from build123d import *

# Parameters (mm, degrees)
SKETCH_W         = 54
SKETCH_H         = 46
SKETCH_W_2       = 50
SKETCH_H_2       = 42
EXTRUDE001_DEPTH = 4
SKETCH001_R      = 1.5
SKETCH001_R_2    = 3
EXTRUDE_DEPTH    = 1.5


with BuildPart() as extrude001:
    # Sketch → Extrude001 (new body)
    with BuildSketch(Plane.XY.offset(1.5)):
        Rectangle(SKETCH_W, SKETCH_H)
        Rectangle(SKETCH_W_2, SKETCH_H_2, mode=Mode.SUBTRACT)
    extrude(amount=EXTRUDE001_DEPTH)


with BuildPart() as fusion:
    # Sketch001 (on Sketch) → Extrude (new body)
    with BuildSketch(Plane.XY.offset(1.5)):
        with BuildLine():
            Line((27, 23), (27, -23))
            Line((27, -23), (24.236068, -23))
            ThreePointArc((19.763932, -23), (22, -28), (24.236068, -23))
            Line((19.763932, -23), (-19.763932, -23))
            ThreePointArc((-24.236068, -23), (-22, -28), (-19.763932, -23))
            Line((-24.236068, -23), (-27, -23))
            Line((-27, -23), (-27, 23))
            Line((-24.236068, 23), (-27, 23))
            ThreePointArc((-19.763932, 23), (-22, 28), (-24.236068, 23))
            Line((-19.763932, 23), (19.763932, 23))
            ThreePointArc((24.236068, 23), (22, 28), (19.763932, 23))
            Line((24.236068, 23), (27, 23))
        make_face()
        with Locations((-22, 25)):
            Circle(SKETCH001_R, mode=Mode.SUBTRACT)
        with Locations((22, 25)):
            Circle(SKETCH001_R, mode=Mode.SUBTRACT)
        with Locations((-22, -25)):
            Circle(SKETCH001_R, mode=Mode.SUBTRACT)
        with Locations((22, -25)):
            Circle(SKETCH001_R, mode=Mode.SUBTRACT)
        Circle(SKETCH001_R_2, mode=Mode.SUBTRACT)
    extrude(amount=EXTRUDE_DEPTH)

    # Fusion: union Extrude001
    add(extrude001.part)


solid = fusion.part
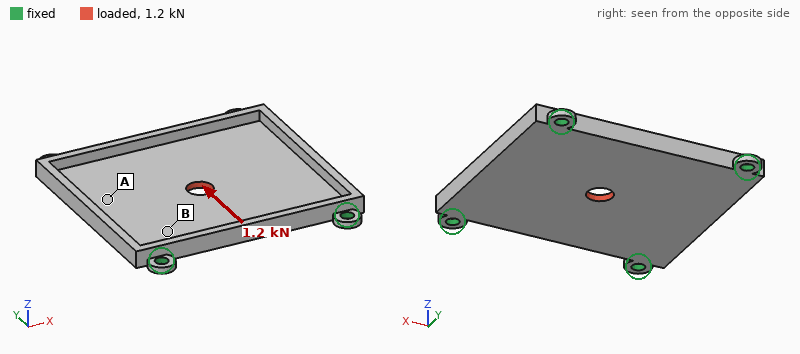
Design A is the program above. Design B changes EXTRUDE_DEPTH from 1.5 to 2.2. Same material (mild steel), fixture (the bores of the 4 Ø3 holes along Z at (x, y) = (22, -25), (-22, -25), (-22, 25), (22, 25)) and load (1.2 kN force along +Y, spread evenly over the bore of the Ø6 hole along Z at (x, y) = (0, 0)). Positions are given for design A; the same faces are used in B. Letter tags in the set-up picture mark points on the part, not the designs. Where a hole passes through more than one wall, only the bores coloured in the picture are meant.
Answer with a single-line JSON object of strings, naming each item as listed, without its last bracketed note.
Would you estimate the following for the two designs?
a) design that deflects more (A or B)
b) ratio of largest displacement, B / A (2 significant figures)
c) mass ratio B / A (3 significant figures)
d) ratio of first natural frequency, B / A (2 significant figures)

{"design that deflects more": "A", "ratio of largest displacement, B / A": "0.69", "mass ratio B / A": "1.32", "ratio of first natural frequency, B / A": "1.2"}
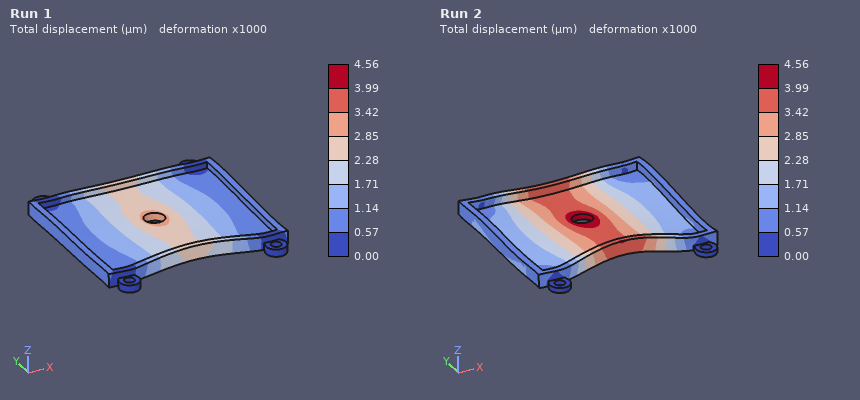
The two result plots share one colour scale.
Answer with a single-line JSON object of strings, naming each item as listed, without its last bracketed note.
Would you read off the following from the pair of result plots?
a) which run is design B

{"which run is design B": "Run 1"}
